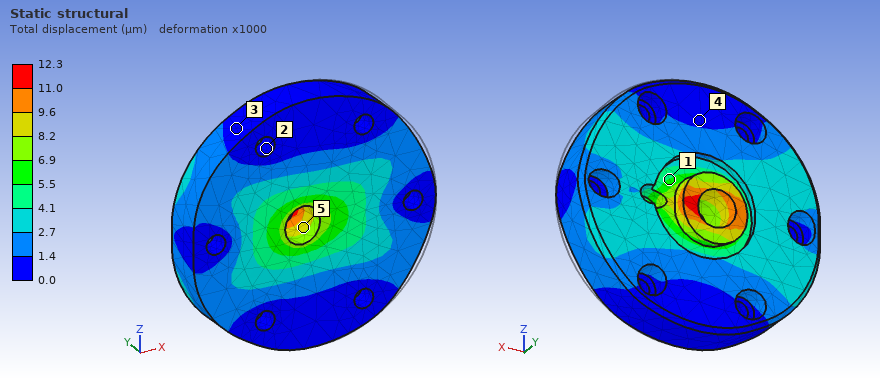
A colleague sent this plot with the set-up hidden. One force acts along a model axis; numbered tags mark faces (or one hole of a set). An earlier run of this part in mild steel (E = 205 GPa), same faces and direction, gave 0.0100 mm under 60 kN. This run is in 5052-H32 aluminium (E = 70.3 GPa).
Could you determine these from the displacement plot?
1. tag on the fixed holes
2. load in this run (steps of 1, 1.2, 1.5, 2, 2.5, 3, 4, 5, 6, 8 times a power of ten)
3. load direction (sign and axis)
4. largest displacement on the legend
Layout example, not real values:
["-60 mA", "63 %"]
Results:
["2", "25 kN", "-X", "12.3 µm"]
